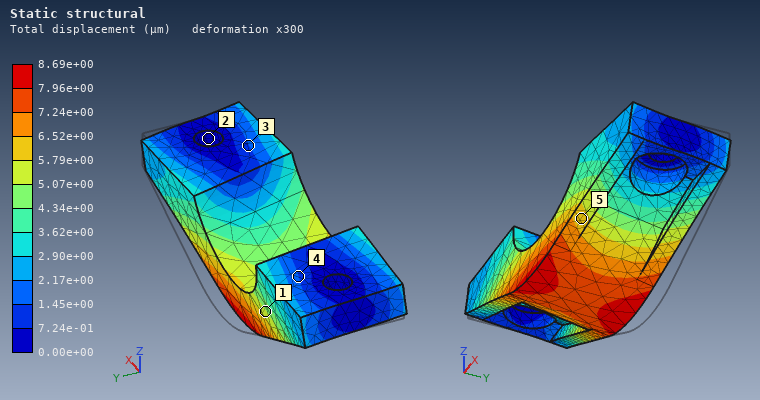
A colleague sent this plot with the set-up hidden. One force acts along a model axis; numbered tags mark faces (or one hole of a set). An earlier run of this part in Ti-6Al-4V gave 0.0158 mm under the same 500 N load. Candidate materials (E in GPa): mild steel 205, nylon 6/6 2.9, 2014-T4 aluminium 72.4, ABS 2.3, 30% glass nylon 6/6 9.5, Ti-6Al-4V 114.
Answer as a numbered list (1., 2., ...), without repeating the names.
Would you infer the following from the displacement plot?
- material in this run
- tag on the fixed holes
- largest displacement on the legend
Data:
1. mild steel
2. 2
3. 8.69e+00 µm
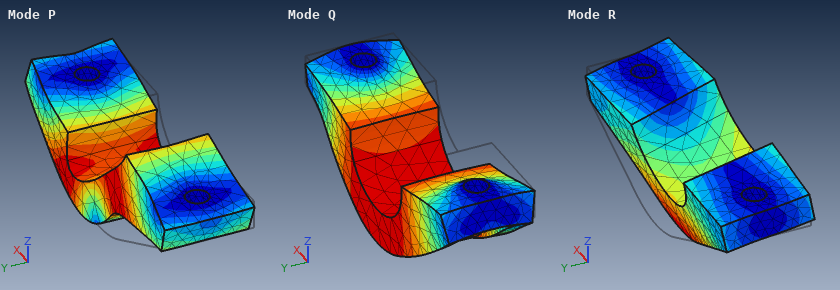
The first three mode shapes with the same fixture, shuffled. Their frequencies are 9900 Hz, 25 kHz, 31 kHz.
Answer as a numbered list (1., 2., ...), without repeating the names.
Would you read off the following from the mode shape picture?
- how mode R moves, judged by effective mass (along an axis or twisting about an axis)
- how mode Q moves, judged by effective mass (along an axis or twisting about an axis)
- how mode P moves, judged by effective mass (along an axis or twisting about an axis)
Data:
1. along Y
2. along Z
3. along X
